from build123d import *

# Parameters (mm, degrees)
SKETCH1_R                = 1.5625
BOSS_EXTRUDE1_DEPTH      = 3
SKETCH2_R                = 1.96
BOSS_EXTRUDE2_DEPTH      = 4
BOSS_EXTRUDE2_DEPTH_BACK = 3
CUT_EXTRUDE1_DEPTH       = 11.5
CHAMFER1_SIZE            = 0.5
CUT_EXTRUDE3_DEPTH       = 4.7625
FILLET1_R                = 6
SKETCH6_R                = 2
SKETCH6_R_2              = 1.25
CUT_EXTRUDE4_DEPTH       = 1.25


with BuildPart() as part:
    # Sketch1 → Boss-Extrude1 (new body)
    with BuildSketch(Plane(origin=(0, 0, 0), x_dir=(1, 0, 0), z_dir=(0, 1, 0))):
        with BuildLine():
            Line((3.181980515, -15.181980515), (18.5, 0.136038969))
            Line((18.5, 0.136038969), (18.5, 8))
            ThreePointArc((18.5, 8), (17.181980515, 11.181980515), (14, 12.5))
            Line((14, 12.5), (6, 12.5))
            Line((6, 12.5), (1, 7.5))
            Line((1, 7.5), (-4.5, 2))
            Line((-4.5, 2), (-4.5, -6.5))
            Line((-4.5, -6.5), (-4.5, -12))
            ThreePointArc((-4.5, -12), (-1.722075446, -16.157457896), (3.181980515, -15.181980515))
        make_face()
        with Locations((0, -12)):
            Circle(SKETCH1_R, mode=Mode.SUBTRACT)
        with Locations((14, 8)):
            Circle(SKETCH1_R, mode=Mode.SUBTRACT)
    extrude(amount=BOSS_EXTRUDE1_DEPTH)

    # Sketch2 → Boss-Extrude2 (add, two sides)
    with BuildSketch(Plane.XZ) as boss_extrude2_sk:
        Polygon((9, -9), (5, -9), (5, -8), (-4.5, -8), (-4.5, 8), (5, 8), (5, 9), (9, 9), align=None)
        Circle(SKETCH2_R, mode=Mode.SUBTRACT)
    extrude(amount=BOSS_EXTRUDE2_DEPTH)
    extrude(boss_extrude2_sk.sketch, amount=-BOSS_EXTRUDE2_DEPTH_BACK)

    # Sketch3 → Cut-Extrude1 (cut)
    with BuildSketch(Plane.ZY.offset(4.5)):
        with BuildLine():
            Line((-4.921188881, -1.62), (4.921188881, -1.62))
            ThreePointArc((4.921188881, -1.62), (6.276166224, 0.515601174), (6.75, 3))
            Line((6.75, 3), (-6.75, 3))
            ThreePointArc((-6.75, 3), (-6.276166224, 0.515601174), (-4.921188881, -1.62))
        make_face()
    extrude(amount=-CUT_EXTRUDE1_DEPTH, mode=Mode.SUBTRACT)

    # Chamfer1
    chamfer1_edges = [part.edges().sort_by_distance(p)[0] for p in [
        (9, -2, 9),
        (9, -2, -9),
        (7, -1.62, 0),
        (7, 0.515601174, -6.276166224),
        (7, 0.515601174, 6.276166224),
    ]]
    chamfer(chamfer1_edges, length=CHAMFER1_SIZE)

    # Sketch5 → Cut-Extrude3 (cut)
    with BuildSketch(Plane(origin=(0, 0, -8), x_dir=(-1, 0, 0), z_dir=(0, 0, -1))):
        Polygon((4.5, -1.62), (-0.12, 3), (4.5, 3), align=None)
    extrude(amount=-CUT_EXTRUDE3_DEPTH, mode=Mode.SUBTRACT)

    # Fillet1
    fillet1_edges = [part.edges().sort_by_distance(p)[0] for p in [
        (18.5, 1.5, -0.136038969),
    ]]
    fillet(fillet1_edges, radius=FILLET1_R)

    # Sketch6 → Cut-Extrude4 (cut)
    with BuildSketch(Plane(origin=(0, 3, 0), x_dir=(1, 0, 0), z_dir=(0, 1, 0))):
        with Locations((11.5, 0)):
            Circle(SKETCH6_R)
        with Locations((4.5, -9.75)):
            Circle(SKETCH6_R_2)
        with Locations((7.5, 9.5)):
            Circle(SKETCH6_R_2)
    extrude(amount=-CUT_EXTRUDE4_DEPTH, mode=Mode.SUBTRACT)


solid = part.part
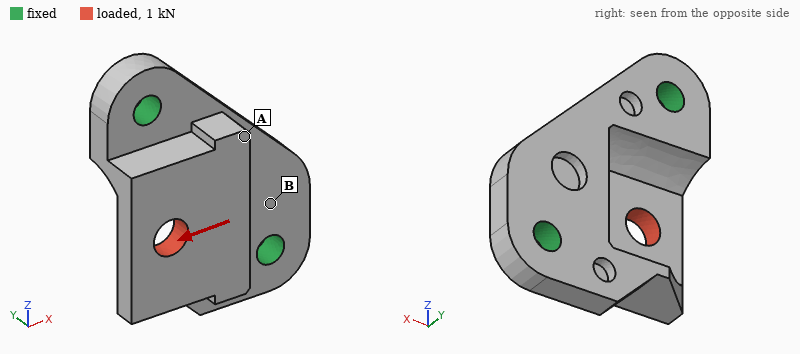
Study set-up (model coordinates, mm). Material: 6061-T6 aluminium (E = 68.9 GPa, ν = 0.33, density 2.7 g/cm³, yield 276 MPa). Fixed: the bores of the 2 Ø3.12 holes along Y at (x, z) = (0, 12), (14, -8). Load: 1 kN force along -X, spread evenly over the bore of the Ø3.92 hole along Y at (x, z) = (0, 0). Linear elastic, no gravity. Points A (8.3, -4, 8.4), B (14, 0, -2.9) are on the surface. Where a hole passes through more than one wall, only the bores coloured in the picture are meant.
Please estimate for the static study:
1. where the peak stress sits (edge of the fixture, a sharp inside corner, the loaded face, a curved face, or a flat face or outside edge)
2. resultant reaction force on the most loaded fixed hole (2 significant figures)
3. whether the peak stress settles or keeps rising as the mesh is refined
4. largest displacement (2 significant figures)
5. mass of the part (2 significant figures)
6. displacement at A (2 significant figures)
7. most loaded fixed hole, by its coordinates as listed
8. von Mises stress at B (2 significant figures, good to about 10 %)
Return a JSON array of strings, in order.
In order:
["edge of the fixture", "610 N", "keeps rising", "79 µm", "4.2 g", "32 µm", "(0, 12)", "43 MPa"]
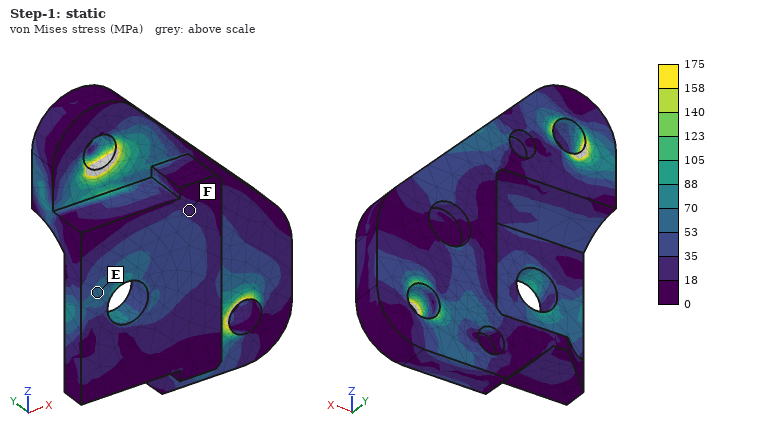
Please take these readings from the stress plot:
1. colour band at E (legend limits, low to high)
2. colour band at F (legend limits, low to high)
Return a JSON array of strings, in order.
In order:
["53 to 70 MPa", "18 to 35 MPa"]
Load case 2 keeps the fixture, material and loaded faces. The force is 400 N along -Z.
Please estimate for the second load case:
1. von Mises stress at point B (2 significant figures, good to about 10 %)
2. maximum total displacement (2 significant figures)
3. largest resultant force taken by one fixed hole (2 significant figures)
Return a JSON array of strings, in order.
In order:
["14 MPa", "16 µm", "260 N"]
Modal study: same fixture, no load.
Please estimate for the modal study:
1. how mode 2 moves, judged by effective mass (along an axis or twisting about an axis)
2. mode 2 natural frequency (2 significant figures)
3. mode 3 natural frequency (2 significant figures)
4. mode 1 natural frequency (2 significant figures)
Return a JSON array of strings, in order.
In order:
["along Y", "24 kHz", "28 kHz", "13 kHz"]
